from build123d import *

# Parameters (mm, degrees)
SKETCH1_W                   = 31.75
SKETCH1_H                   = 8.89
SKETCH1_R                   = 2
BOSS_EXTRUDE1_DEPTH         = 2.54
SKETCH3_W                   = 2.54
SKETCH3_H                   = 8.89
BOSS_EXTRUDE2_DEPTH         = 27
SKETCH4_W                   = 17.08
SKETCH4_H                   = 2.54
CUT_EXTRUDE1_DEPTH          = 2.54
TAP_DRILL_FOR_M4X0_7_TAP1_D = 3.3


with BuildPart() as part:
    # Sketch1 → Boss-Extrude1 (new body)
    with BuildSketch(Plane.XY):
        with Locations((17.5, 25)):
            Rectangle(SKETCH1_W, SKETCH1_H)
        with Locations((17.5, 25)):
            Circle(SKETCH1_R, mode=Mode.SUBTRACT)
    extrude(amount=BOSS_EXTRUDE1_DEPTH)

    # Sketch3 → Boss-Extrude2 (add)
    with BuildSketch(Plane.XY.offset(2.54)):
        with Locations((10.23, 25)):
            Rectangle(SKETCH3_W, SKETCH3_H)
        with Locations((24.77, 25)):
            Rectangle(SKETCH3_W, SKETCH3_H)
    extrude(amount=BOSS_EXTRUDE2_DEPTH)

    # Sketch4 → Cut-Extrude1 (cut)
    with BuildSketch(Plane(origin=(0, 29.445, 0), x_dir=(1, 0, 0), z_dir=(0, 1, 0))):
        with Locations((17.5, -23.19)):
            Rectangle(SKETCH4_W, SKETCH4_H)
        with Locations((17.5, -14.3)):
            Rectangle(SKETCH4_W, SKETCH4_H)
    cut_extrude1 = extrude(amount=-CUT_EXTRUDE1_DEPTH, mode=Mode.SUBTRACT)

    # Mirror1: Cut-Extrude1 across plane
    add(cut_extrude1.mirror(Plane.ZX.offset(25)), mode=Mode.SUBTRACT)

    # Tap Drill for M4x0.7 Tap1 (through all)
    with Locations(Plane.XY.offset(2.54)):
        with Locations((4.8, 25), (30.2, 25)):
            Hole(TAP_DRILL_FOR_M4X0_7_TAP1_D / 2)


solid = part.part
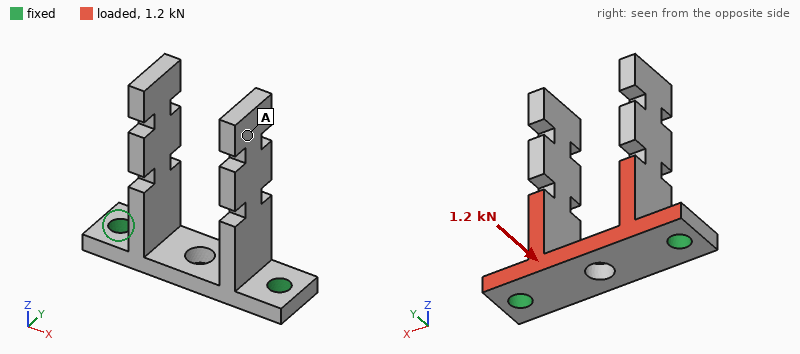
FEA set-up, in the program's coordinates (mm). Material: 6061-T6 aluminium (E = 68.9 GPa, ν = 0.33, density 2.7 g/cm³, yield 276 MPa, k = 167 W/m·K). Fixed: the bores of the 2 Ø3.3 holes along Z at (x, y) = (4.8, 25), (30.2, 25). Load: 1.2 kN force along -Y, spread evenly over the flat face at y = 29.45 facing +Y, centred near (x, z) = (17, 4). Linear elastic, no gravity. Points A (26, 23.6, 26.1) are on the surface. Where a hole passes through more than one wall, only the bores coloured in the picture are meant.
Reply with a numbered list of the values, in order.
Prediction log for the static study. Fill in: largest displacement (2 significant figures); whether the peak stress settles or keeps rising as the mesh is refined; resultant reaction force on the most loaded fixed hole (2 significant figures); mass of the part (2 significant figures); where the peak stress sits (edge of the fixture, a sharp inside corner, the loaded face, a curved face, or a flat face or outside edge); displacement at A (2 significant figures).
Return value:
1. 0.14 mm
2. keeps rising
3. 600 N
4. 4.7 g
5. edge of the fixture
6. 0.12 mm
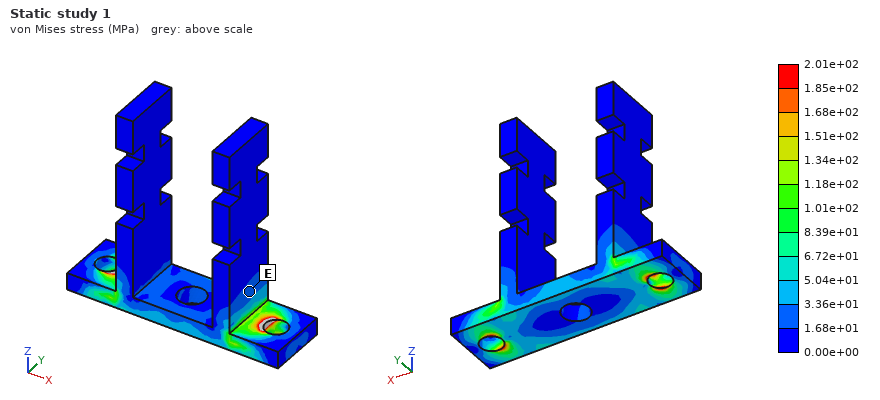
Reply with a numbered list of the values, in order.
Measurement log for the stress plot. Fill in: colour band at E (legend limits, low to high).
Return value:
1. 1.68e+01 to 3.36e+01 MPa
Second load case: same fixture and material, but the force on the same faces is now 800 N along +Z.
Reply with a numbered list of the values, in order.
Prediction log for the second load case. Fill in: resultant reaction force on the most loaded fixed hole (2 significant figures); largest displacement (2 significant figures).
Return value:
1. 400 N
2. 0.16 mm
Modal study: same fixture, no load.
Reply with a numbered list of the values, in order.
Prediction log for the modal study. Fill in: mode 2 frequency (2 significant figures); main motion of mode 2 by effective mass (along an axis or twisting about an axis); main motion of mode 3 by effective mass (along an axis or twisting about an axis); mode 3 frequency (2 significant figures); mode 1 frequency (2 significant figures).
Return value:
1. 2500 Hz
2. along X
3. along Y
4. 3800 Hz
5. 2300 Hz
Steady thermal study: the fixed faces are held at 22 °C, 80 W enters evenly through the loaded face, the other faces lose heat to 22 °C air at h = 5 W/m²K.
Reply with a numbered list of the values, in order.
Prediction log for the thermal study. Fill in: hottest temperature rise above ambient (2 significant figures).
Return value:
1. 71 K
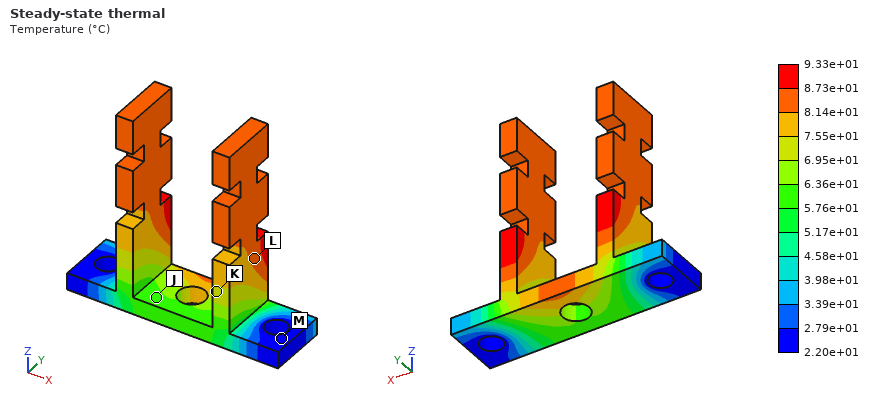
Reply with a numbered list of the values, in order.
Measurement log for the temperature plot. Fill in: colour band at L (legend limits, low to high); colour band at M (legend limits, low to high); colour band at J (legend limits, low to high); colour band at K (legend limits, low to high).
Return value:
1. 8.14e+01 to 8.73e+01 °C
2. 2.20e+01 to 2.79e+01 °C
3. 5.76e+01 to 6.36e+01 °C
4. 6.95e+01 to 7.55e+01 °C
